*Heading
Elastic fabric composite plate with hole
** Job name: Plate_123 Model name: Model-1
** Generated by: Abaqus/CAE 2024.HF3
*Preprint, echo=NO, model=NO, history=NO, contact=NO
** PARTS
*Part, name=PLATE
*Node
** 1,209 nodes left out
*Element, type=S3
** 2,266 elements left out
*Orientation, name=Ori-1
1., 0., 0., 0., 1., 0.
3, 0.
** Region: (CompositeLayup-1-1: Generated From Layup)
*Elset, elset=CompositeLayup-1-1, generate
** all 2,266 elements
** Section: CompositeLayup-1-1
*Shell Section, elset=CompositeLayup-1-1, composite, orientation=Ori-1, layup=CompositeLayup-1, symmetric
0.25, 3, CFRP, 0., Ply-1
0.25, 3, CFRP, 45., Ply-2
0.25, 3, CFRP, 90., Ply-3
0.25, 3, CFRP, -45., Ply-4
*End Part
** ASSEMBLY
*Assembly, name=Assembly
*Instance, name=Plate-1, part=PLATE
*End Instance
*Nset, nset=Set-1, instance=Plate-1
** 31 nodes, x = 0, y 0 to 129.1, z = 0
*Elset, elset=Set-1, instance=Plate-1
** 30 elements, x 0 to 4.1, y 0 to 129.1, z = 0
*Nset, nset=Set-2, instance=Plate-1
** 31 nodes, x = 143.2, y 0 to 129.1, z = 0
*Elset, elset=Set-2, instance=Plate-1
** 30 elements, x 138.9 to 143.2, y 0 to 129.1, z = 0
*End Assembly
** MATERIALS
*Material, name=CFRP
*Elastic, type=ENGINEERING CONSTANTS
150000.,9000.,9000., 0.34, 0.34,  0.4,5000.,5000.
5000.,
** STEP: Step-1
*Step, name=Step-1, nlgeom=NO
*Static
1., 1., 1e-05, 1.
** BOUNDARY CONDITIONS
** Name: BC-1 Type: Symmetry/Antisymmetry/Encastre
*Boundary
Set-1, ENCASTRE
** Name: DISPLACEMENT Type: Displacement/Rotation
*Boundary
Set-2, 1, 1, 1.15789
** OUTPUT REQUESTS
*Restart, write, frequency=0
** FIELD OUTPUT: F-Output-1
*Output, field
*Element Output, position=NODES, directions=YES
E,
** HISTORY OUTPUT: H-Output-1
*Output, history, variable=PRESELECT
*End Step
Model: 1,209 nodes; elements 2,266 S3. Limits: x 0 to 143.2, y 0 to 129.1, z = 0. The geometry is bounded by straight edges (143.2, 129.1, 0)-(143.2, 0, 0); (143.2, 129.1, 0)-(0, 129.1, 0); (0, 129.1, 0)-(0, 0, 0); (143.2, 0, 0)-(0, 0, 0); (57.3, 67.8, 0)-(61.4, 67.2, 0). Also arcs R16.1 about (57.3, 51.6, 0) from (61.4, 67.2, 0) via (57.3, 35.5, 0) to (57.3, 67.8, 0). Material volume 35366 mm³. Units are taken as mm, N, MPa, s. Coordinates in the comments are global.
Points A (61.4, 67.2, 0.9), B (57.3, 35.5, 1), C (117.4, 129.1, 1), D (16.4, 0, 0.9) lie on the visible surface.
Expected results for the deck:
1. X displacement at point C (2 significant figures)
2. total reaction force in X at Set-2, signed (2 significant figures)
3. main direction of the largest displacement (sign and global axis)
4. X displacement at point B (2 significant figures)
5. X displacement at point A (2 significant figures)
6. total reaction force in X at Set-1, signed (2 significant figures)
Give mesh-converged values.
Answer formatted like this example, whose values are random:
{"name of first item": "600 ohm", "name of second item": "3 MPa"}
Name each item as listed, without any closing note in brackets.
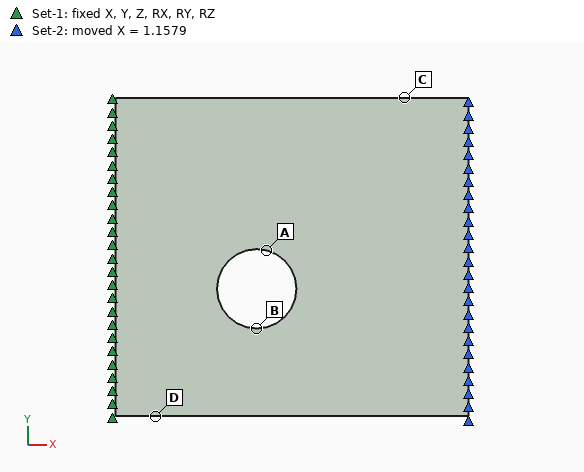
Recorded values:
{"X displacement at point C": "0.94 mm", "total reaction force in X at Set-2, signed": "1.1e+05 N", "main direction of the largest displacement": "+X", "X displacement at point B": "0.47 mm", "X displacement at point A": "0.57 mm", "total reaction force in X at Set-1, signed": "-1.1e+05 N"}
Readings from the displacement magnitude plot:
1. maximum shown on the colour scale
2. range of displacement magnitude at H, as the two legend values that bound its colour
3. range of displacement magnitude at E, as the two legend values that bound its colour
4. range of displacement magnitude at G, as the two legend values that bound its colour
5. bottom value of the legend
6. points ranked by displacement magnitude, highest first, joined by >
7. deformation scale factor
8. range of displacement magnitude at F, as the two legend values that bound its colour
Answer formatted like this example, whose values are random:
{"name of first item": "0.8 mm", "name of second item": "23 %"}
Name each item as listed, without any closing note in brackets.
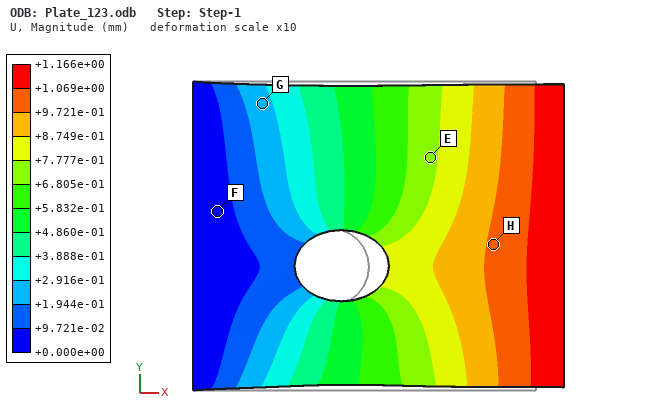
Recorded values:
{"maximum shown on the colour scale": "+1.166e+00 mm", "range of displacement magnitude at H, as the two legend values that bound its colour": "+9.721e-01 to +1.069e+00 mm", "range of displacement magnitude at E, as the two legend values that bound its colour": "+6.805e-01 to +7.777e-01 mm", "range of displacement magnitude at G, as the two legend values that bound its colour": "+1.944e-01 to +2.916e-01 mm", "bottom value of the legend": "+0.000e+00 mm", "points ranked by displacement magnitude, highest first, joined by >": "H > E > G > F", "deformation scale factor": "10", "range of displacement magnitude at F, as the two legend values that bound its colour": "+0.000e+00 to +9.721e-02 mm"}
